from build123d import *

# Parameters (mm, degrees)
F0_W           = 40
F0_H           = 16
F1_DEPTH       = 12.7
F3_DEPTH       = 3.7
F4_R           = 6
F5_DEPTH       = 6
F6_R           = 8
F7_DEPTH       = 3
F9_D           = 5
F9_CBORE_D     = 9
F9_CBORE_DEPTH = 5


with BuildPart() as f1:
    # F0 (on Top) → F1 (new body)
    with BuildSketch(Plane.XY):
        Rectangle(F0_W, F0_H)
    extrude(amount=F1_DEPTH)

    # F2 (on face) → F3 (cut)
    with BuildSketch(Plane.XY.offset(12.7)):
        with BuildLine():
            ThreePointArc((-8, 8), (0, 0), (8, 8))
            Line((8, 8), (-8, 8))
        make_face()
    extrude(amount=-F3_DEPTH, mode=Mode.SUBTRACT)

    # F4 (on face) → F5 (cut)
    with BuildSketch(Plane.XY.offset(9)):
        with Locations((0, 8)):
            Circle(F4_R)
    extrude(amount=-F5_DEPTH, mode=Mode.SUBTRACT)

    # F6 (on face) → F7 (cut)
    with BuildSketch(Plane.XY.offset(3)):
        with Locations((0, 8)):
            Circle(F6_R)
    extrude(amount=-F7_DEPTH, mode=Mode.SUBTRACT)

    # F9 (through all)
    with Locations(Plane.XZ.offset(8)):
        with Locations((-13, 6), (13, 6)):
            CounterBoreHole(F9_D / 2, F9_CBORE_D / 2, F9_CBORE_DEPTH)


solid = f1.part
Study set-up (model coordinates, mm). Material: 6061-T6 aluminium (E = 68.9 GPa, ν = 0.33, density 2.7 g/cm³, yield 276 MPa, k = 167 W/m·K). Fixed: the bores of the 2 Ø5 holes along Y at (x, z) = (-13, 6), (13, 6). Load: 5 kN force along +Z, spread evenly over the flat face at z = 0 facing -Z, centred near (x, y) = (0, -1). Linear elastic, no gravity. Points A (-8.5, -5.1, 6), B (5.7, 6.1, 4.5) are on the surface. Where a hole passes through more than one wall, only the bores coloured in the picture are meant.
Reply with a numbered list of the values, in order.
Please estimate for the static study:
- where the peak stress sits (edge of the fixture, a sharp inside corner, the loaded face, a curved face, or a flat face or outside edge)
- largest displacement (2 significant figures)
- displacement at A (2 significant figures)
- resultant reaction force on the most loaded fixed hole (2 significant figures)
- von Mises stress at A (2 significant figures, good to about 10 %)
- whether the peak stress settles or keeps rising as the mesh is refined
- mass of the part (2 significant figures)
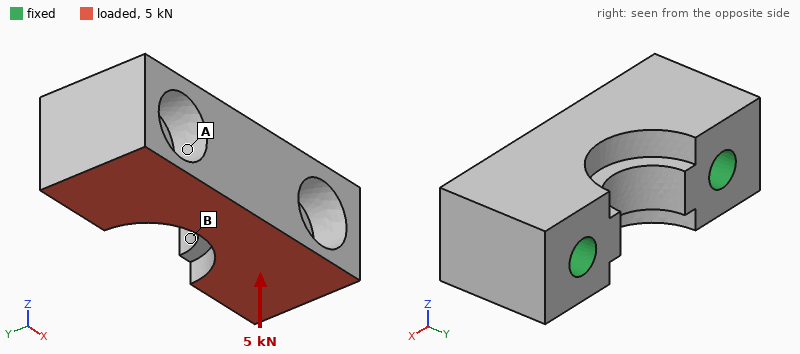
1. edge of the fixture
2. 11 µm
3. 5.2 µm
4. 2.5 kN
5. 30 MPa
6. keeps rising
7. 16 g
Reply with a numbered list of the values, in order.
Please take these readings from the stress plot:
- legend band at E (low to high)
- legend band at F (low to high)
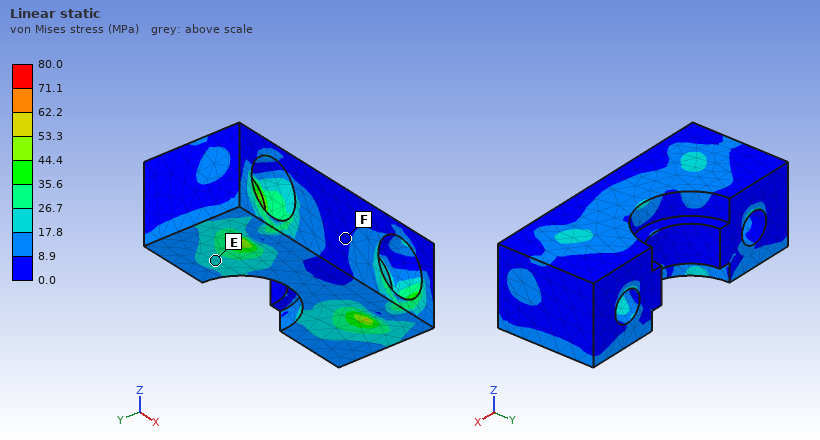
1. 17.8 to 26.7 MPa
2. 0.0 to 8.9 MPa
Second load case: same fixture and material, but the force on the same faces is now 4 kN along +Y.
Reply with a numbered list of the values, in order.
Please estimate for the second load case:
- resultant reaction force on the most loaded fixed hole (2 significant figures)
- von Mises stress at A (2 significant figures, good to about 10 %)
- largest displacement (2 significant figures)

1. 2.0 kN
2. 17 MPa
3. 10 µm
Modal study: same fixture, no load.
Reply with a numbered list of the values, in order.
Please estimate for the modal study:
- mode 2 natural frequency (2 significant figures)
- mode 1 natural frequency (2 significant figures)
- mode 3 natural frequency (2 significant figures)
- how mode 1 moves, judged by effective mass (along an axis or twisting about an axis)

1. 54 kHz
2. 35 kHz
3. 56 kHz
4. along Z
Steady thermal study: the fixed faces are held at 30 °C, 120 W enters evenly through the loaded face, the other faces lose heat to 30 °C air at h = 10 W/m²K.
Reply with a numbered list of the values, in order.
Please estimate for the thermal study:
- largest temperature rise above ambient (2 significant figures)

1. 18 K
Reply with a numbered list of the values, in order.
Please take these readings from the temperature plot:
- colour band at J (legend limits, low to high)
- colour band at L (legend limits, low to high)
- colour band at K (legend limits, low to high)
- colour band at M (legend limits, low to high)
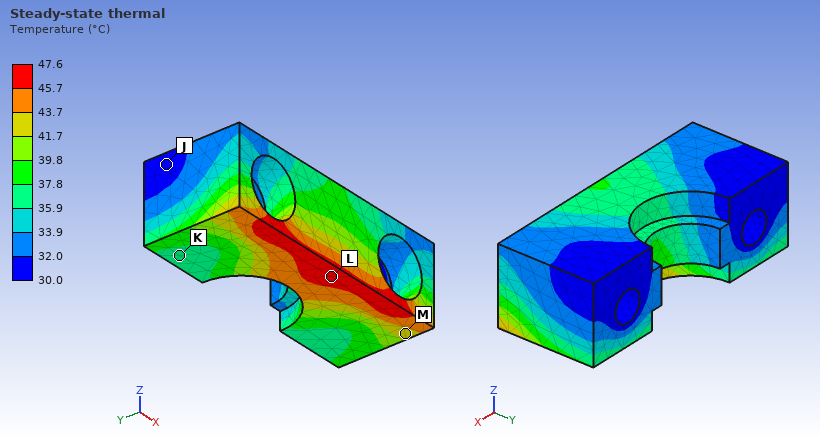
1. 30.0 to 32.0 °C
2. 45.7 to 47.6 °C
3. 35.9 to 37.8 °C
4. 41.7 to 43.7 °C
